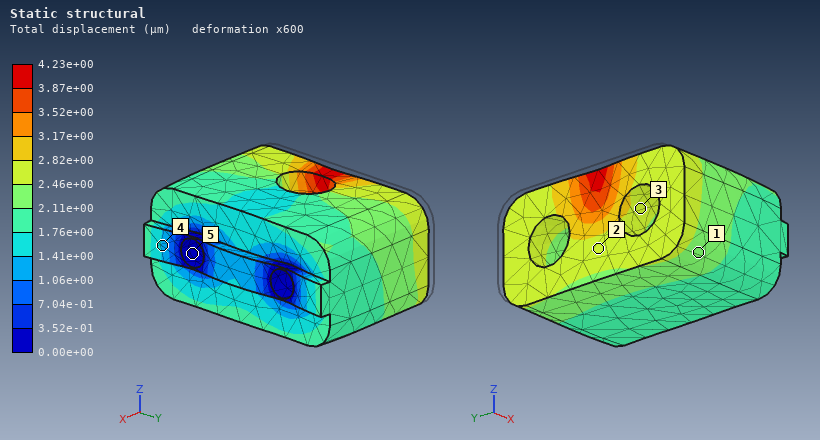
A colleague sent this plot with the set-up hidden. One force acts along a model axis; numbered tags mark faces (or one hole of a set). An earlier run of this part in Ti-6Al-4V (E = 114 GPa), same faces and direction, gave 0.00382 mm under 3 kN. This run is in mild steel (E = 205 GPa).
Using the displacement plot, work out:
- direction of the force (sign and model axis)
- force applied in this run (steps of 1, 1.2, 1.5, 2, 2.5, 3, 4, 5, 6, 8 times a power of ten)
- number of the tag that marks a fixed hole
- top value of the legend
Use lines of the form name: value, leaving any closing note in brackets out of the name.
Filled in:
direction of the force: +X
force applied in this run: 6 kN
number of the tag that marks a fixed hole: 5
top value of the legend: 4.23e+00 µm
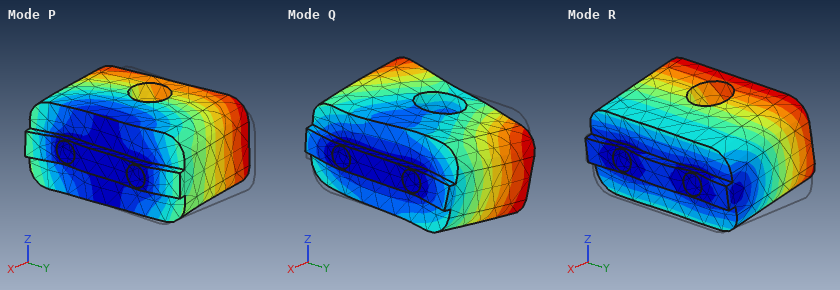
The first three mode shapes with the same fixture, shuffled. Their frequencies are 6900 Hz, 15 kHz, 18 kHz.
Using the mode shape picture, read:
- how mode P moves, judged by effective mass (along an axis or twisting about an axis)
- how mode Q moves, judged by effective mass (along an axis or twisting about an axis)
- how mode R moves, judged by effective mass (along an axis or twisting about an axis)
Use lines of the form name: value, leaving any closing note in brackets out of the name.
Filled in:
how mode P moves, judged by effective mass: along Y
how mode Q moves, judged by effective mass: twisting about X
how mode R moves, judged by effective mass: along Z
